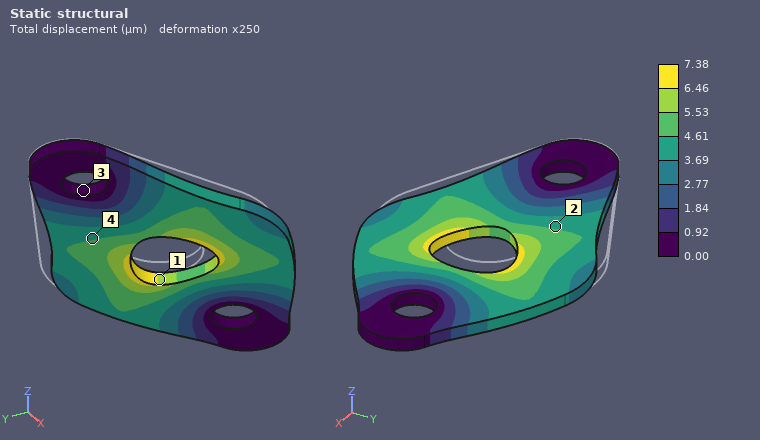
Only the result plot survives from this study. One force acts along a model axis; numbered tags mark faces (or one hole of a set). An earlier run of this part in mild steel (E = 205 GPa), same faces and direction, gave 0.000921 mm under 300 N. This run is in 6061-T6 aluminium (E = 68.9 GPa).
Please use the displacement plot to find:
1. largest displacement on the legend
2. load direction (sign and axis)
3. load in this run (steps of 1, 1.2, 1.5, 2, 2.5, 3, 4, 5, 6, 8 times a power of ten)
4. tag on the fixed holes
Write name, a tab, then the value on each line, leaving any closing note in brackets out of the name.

largest displacement on the legend	7.38 µm
load direction	+X
load in this run	800 N
tag on the fixed holes	3
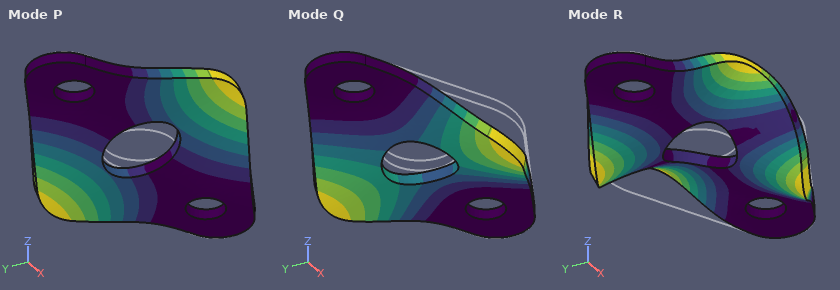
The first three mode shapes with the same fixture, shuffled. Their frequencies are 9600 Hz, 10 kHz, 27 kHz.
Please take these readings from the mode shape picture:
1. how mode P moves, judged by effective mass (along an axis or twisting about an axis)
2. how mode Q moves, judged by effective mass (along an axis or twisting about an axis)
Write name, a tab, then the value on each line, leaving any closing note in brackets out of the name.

how mode P moves, judged by effective mass	twisting about X
how mode Q moves, judged by effective mass	along Z
